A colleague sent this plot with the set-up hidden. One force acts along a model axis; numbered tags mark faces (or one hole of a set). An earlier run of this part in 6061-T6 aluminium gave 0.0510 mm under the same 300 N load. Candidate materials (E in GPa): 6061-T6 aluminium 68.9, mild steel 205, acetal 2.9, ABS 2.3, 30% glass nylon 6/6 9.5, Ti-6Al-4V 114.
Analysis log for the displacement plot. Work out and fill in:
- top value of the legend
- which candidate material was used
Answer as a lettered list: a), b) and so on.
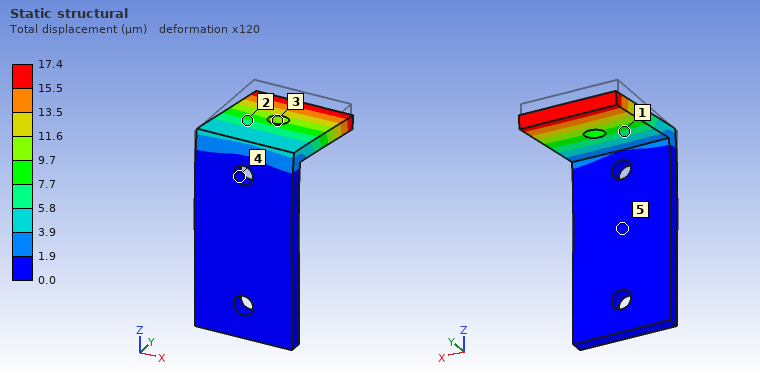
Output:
a) 17.4 µm
b) mild steel
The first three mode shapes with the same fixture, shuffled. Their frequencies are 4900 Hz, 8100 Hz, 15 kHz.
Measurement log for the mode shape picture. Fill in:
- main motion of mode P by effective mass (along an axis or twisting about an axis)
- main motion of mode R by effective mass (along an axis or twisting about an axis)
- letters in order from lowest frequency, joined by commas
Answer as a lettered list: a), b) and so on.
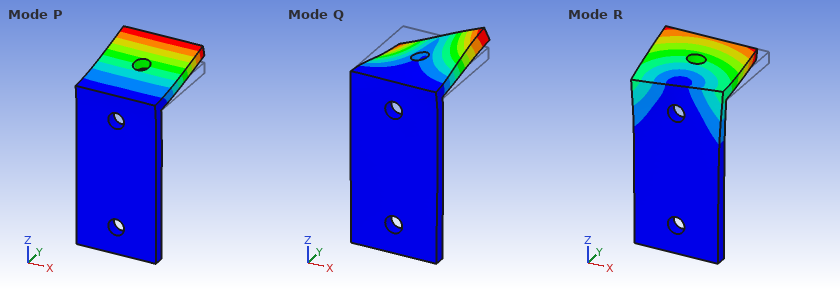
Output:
a) along Z
b) along X
c) P, R, Q
